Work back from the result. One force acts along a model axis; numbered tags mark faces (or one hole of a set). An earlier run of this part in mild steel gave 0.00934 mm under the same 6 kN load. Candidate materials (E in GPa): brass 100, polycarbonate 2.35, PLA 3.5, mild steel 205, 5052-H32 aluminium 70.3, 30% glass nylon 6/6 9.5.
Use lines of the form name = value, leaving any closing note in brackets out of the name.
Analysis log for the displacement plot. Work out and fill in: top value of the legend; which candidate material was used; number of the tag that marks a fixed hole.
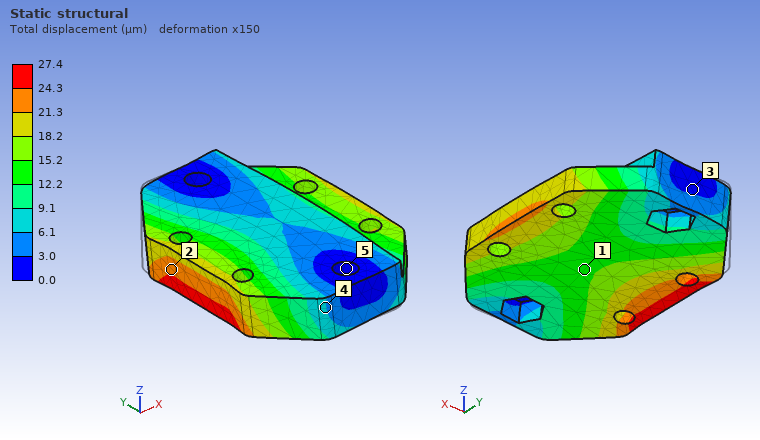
top value of the legend = 27.4 µm
which candidate material was used = 5052-H32 aluminium
number of the tag that marks a fixed hole = 5
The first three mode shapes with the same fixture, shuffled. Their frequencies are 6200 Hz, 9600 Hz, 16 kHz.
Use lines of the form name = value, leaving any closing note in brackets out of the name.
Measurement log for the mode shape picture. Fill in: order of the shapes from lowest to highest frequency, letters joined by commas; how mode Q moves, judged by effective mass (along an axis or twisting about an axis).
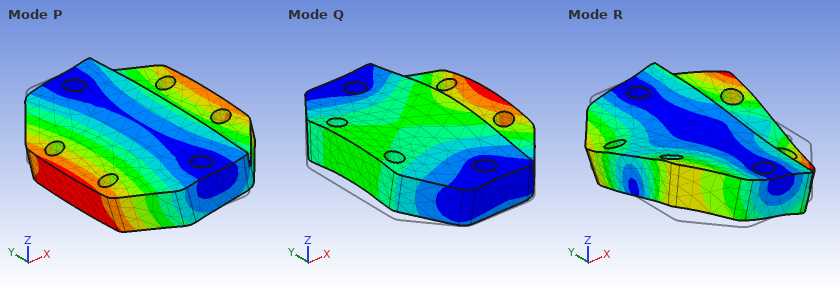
order of the shapes from lowest to highest frequency, letters joined by commas = P, Q, R
how mode Q moves, judged by effective mass = along Z
